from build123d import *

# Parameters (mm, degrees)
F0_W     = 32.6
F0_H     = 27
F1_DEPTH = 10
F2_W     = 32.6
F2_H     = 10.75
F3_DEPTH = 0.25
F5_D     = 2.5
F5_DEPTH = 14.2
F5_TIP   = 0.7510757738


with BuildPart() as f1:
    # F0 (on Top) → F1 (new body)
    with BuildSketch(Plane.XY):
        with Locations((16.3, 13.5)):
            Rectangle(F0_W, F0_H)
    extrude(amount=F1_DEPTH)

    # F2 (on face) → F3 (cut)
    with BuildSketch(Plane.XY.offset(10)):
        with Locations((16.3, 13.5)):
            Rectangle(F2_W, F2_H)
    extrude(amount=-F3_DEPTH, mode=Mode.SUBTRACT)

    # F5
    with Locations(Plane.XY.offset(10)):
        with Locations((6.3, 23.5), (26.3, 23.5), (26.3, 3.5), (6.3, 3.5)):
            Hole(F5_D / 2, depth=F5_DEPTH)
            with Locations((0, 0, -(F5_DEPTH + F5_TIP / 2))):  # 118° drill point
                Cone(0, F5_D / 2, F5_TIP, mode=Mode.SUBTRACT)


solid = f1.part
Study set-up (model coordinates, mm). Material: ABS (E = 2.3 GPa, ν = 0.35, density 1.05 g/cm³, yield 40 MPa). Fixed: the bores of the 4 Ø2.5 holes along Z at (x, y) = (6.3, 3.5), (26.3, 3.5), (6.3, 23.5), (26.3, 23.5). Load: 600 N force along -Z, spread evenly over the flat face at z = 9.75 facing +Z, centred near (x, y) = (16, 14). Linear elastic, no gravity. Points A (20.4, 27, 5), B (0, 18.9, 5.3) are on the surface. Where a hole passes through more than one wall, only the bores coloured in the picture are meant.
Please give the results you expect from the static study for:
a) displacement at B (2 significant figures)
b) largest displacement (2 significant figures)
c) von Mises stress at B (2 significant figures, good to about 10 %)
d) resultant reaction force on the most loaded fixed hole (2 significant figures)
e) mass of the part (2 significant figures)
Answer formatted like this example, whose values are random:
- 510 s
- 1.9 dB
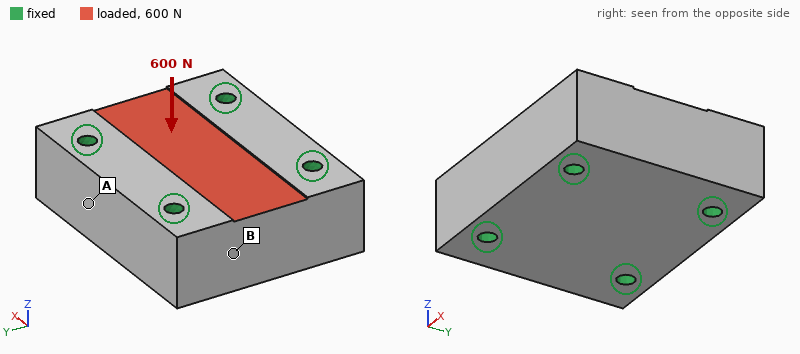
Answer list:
- 11 µm
- 20 µm
- 2.2 MPa
- 150 N
- 8.9 g
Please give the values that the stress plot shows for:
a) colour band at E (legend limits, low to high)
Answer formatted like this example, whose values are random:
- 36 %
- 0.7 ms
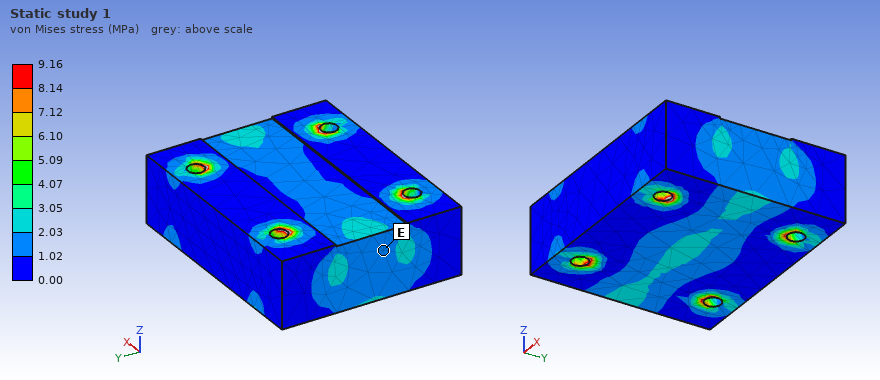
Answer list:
- 1.02 to 2.03 MPa
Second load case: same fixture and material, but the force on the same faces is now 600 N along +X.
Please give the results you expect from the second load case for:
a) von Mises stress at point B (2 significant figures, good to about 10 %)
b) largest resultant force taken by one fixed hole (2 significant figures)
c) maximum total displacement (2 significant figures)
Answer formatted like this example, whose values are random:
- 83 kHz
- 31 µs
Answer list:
- 2.6 MPa
- 160 N
- 31 µm
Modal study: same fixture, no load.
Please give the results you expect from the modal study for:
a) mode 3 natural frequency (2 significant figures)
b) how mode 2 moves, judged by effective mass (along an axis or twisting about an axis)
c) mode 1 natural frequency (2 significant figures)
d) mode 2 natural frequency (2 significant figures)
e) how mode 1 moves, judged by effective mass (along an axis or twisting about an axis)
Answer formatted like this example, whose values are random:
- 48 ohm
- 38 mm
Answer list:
- 18 kHz
- twisting about Y
- 14 kHz
- 17 kHz
- along Z
